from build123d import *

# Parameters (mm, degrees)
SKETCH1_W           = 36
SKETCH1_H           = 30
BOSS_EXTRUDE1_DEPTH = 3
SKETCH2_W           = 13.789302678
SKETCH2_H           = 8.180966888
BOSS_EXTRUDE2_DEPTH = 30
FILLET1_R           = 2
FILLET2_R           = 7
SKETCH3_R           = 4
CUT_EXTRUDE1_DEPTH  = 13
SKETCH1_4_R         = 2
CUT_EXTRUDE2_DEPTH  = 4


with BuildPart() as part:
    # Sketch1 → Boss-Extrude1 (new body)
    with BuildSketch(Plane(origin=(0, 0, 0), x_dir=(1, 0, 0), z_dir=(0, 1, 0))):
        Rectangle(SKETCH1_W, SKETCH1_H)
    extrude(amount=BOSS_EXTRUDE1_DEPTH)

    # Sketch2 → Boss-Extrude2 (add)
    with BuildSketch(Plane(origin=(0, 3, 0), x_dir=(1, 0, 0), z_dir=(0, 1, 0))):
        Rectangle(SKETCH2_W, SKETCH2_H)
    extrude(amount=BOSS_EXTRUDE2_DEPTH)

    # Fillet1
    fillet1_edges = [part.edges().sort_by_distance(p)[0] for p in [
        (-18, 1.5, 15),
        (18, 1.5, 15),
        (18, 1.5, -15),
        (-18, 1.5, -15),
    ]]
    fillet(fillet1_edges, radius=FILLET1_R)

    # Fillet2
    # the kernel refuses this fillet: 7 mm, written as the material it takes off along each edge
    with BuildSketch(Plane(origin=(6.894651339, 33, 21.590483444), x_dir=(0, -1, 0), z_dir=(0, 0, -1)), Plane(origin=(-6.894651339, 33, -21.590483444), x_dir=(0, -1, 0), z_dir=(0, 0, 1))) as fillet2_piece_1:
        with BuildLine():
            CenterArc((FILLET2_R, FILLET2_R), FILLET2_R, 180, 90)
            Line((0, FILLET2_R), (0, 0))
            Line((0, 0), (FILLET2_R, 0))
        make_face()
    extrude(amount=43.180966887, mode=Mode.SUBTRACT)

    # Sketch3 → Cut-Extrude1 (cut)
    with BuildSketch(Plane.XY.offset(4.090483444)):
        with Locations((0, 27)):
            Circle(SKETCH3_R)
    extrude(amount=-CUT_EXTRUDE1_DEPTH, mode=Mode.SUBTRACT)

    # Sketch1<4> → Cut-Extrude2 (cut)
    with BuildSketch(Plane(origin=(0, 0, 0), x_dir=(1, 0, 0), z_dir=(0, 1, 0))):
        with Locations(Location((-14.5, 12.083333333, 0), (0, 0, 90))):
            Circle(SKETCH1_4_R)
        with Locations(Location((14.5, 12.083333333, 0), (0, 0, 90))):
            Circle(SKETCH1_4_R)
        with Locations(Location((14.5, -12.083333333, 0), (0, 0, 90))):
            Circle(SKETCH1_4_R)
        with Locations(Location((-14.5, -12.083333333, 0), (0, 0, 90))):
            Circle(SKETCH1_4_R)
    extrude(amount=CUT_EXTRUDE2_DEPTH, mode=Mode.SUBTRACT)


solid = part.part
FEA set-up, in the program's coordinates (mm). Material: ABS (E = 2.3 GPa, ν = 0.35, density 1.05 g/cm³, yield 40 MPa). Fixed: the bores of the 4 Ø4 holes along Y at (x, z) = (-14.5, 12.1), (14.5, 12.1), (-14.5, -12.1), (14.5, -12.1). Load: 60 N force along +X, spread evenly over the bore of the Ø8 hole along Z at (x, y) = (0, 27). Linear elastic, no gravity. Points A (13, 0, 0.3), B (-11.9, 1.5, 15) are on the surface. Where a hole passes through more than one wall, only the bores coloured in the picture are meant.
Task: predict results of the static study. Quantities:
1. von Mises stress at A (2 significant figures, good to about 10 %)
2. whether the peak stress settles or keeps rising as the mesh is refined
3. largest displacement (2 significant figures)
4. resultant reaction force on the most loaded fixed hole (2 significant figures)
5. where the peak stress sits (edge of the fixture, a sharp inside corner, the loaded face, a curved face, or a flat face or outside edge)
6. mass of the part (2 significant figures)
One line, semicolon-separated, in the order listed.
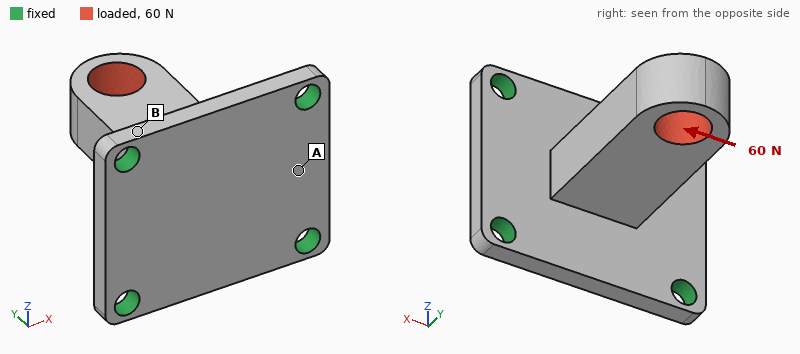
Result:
4.3 MPa; keeps rising; 0.44 mm; 37 N; edge of the fixture; 6.2 g
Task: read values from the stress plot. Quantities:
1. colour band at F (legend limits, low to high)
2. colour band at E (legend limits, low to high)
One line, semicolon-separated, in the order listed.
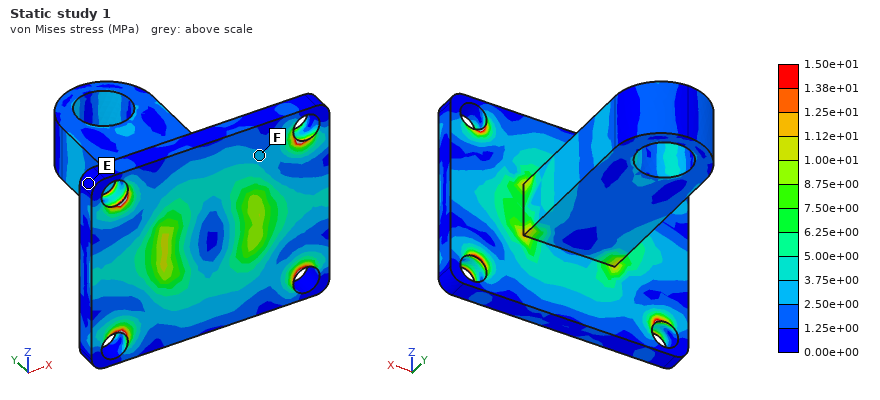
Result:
2.50e+00 to 3.75e+00 MPa; 0.00e+00 to 1.25e+00 MPa
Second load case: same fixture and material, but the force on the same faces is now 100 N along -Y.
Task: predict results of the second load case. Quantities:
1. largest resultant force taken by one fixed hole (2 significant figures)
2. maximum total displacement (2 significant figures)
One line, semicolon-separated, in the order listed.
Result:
26 N; 94 µm
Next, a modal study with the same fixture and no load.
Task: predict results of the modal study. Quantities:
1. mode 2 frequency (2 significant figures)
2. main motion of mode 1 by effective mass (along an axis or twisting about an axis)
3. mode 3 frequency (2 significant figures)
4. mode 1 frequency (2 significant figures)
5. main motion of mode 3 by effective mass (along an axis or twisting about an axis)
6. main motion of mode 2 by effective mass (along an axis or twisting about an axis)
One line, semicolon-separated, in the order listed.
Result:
1900 Hz; along Z; 2900 Hz; 1500 Hz; along Y; along X
